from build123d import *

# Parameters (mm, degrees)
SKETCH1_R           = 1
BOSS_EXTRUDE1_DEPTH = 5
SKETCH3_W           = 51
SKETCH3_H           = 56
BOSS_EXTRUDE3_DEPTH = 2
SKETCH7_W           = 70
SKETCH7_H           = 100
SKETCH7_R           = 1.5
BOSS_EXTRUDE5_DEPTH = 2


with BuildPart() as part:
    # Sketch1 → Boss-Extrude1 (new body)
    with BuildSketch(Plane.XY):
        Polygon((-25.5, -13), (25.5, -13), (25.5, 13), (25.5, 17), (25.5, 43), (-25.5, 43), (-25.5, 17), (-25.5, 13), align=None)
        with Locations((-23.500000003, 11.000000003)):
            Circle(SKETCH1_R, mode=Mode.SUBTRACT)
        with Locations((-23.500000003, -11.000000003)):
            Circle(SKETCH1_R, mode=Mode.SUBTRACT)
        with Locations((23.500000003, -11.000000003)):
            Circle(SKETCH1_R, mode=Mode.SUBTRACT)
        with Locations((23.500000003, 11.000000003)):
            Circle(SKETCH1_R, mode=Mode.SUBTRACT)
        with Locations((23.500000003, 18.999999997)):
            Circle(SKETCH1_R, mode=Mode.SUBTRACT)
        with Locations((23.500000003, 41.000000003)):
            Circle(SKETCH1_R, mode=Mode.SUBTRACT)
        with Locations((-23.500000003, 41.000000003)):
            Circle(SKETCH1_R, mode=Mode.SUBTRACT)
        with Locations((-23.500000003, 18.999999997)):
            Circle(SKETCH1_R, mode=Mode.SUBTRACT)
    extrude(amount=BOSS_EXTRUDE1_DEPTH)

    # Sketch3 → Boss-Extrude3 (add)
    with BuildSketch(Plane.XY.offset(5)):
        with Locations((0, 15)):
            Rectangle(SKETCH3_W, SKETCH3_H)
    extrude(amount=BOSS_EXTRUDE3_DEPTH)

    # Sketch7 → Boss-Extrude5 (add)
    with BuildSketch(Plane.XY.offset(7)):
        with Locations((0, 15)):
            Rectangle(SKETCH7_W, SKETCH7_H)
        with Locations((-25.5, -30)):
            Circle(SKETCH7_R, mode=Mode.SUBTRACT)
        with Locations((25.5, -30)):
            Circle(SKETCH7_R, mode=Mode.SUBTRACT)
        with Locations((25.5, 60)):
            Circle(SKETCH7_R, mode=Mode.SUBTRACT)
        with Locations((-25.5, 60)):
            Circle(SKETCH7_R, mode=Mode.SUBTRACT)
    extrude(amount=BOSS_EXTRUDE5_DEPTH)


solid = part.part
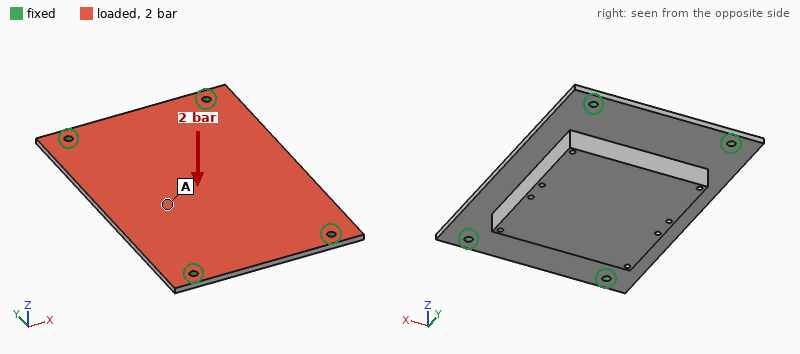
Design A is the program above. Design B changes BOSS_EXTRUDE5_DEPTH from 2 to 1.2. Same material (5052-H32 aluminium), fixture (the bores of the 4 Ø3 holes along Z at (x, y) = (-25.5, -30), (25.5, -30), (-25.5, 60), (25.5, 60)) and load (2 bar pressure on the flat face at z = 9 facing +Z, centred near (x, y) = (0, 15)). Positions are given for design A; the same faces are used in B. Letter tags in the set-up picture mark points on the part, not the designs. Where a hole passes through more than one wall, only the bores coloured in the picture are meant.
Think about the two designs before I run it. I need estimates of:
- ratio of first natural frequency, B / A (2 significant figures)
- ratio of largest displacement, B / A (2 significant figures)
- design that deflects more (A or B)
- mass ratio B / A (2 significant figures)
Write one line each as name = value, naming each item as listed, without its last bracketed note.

ratio of first natural frequency, B / A = 0.56
ratio of largest displacement, B / A = 3.6
design that deflects more = B
mass ratio B / A = 0.84
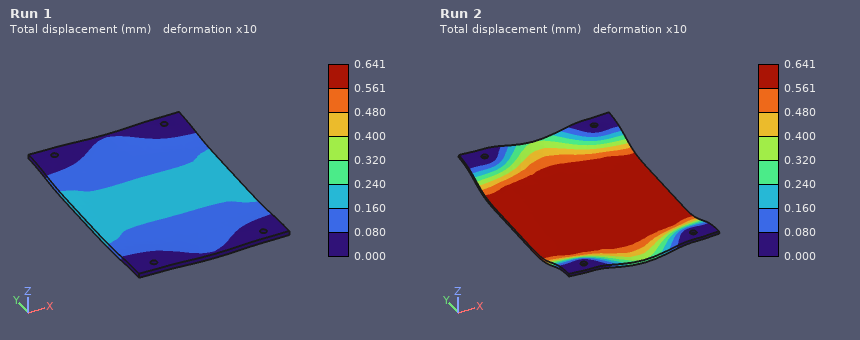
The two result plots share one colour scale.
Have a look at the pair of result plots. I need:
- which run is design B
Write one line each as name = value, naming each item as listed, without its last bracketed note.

which run is design B = Run 2
